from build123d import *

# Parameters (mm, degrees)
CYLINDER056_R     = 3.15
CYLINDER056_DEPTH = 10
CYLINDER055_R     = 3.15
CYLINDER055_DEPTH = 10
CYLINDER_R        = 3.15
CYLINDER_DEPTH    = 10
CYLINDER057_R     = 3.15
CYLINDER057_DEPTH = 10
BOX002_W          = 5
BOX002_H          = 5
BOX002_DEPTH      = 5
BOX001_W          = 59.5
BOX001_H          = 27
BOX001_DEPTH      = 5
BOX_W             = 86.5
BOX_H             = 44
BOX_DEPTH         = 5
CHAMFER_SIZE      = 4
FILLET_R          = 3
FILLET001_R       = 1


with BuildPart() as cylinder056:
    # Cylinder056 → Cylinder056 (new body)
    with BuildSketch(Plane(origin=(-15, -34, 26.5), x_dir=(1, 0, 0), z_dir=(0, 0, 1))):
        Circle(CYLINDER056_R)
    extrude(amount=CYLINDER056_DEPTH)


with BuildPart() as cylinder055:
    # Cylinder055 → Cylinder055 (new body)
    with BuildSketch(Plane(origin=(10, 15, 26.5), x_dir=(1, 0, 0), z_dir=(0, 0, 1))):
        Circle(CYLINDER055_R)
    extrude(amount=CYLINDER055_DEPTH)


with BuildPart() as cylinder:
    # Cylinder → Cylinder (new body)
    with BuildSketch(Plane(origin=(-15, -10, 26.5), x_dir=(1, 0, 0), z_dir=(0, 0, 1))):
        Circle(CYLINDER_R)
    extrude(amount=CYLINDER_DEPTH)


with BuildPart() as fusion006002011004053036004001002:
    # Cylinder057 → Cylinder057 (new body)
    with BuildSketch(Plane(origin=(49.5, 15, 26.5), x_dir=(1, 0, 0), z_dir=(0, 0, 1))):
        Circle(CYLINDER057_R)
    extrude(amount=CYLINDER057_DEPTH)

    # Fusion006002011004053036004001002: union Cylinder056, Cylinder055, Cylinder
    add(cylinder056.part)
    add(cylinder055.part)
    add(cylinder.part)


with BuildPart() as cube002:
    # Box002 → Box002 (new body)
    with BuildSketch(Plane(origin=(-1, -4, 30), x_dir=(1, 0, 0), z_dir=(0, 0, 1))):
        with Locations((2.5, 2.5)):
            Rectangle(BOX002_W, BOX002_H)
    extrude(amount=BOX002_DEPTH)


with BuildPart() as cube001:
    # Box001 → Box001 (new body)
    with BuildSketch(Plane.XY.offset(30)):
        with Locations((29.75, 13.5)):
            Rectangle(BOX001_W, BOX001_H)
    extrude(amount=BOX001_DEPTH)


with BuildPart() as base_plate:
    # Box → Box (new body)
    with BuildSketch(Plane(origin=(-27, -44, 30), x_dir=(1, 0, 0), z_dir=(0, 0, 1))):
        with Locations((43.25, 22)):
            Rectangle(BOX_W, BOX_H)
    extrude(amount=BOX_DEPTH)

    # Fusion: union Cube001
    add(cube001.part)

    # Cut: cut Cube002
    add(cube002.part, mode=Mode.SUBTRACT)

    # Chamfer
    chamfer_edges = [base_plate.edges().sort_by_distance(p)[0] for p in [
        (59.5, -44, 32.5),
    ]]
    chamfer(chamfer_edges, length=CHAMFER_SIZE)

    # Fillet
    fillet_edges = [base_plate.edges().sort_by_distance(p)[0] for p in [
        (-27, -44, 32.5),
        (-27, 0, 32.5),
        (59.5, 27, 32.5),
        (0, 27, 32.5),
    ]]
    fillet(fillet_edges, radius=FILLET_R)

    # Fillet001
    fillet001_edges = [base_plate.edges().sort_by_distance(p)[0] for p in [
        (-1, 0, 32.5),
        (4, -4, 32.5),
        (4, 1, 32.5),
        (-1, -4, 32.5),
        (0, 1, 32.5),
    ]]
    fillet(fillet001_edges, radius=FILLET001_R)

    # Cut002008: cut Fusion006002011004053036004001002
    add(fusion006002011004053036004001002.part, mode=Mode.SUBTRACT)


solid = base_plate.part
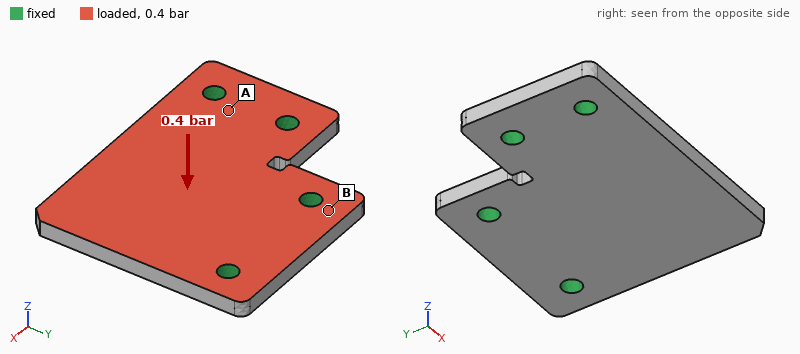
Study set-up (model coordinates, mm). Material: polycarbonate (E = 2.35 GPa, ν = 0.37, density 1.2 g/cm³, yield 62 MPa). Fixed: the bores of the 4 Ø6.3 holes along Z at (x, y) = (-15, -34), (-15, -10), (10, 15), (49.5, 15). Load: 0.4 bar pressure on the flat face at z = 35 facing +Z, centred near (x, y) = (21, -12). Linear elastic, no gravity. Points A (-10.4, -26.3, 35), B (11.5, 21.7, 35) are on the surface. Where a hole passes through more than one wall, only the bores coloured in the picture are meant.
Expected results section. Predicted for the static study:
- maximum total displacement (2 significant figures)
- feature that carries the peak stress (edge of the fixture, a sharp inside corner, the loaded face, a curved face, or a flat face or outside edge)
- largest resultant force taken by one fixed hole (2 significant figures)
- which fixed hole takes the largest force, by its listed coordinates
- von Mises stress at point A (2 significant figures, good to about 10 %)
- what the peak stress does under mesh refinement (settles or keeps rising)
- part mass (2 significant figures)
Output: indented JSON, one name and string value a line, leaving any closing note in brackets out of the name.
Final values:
{
  "maximum total displacement": "1.2 mm",
  "feature that carries the peak stress": "edge of the fixture",
  "largest resultant force taken by one fixed hole": "82 N",
  "which fixed hole takes the largest force, by its listed coordinates": "(49.5, 15)",
  "von Mises stress at point A": "4.3 MPa",
  "what the peak stress does under mesh refinement": "keeps rising",
  "part mass": "31 g"
}
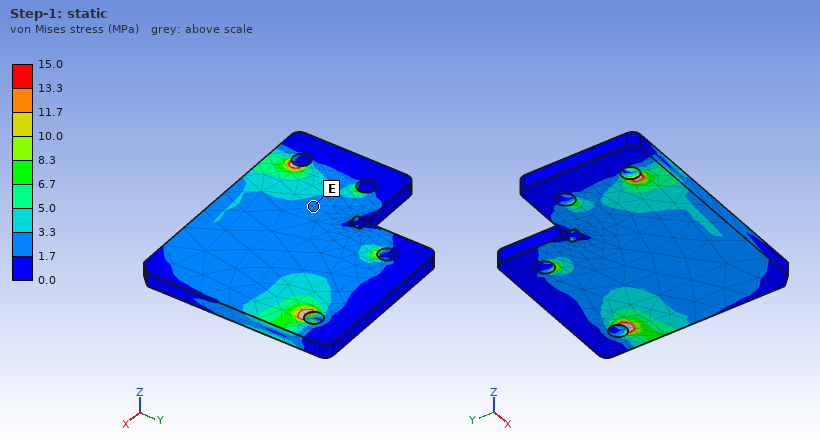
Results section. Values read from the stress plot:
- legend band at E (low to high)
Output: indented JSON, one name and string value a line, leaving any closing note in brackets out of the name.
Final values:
{
  "legend band at E": "1.7 to 3.3 MPa"
}
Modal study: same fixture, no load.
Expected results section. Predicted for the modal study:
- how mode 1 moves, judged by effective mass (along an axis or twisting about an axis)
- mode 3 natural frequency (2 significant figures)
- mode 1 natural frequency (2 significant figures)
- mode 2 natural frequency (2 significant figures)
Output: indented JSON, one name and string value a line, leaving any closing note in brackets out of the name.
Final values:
{
  "how mode 1 moves, judged by effective mass": "along Z",
  "mode 3 natural frequency": "2200 Hz",
  "mode 1 natural frequency": "540 Hz",
  "mode 2 natural frequency": "1600 Hz"
}
